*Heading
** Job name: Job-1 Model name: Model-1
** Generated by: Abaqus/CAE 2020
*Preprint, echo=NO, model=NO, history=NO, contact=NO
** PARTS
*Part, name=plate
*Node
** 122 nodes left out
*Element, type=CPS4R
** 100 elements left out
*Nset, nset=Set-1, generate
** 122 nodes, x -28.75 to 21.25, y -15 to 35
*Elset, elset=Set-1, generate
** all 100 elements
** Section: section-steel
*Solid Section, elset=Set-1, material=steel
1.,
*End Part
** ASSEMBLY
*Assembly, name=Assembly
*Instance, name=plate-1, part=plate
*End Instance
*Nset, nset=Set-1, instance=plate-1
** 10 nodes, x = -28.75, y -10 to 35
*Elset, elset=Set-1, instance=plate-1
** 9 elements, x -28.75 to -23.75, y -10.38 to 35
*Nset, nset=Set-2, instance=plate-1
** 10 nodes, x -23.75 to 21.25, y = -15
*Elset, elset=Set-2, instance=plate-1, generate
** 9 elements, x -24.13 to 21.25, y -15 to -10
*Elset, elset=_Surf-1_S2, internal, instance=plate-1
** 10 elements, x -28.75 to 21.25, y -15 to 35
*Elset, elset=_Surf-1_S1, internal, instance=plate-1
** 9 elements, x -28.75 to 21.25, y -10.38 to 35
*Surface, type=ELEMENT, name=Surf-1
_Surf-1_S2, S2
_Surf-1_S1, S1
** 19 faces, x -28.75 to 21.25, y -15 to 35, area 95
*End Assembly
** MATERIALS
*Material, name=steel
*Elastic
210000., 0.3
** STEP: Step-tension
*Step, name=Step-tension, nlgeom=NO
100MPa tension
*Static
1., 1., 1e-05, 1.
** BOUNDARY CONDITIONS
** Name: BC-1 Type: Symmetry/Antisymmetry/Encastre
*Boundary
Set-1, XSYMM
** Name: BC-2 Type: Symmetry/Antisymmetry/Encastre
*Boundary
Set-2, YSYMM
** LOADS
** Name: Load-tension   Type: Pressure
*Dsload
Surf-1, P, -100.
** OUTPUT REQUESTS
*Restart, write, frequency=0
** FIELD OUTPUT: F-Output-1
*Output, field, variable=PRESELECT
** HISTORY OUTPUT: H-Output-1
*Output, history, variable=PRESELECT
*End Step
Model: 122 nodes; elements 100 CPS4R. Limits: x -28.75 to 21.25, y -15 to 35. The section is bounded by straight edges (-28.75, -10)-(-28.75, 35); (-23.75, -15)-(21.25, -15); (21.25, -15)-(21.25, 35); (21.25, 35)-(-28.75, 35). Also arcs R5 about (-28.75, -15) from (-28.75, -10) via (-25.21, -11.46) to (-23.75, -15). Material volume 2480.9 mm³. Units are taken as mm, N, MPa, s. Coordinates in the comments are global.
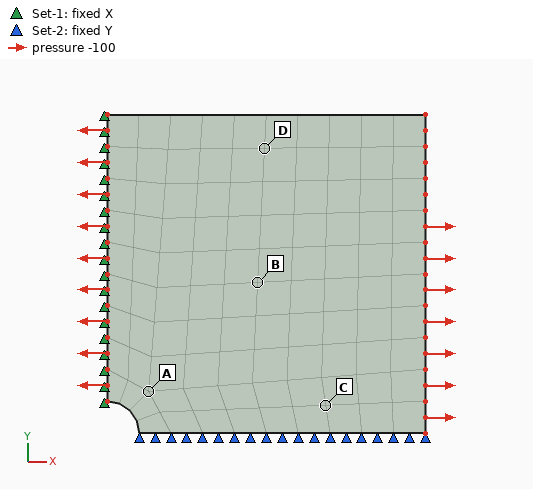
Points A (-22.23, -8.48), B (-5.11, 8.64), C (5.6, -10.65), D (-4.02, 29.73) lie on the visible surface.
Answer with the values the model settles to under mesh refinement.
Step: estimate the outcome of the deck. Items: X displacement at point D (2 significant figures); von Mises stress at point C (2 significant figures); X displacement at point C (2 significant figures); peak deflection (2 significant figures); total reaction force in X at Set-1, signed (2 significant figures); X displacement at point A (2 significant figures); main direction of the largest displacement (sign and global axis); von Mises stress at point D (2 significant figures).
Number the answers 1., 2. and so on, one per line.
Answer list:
1. 0.012 mm
2. 97 MPa
3. 0.018 mm
4. 0.025 mm
5. -500 N
6. 0.0046 mm
7. +X
8. 100 MPa
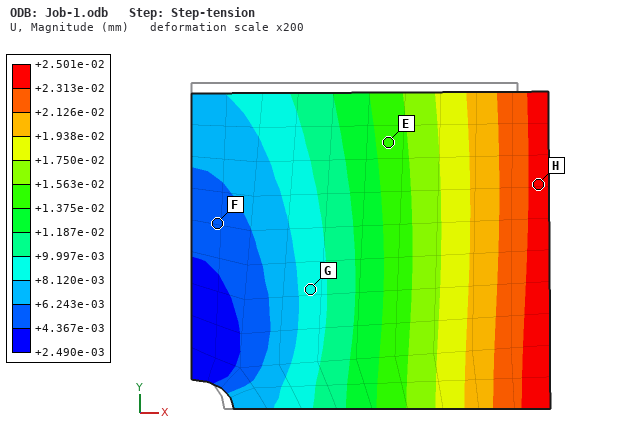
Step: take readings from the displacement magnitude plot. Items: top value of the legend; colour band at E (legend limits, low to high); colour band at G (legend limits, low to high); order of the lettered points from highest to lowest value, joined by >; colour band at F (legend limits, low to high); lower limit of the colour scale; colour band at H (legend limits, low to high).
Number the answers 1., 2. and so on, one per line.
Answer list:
1. +2.501e-02 mm
2. +1.375e-02 to +1.563e-02 mm
3. +8.120e-03 to +9.997e-03 mm
4. H > E > G > F
5. +4.367e-03 to +6.243e-03 mm
6. +2.490e-03 mm
7. +2.313e-02 to +2.501e-02 mm
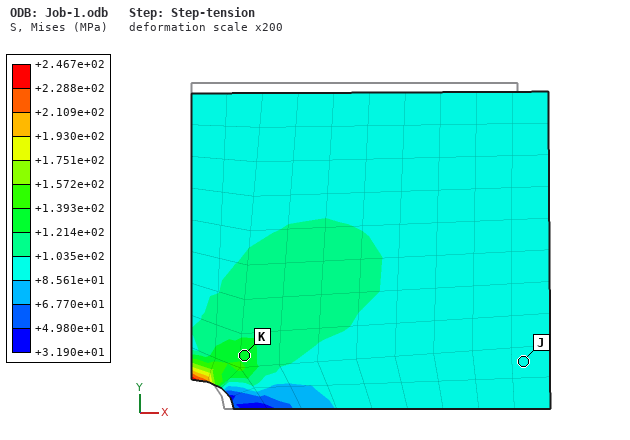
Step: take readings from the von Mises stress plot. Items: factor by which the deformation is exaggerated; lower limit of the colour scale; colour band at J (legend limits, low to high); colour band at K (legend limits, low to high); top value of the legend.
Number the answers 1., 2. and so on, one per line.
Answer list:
1. 200
2. +3.190e+01 MPa
3. +8.561e+01 to +1.035e+02 MPa
4. +1.214e+02 to +1.393e+02 MPa
5. +2.467e+02 MPa
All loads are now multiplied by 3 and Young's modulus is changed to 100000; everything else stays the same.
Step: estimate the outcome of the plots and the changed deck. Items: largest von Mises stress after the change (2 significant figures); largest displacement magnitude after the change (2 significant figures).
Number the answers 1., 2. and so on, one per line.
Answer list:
1. 740 MPa
2. 0.16 mm
